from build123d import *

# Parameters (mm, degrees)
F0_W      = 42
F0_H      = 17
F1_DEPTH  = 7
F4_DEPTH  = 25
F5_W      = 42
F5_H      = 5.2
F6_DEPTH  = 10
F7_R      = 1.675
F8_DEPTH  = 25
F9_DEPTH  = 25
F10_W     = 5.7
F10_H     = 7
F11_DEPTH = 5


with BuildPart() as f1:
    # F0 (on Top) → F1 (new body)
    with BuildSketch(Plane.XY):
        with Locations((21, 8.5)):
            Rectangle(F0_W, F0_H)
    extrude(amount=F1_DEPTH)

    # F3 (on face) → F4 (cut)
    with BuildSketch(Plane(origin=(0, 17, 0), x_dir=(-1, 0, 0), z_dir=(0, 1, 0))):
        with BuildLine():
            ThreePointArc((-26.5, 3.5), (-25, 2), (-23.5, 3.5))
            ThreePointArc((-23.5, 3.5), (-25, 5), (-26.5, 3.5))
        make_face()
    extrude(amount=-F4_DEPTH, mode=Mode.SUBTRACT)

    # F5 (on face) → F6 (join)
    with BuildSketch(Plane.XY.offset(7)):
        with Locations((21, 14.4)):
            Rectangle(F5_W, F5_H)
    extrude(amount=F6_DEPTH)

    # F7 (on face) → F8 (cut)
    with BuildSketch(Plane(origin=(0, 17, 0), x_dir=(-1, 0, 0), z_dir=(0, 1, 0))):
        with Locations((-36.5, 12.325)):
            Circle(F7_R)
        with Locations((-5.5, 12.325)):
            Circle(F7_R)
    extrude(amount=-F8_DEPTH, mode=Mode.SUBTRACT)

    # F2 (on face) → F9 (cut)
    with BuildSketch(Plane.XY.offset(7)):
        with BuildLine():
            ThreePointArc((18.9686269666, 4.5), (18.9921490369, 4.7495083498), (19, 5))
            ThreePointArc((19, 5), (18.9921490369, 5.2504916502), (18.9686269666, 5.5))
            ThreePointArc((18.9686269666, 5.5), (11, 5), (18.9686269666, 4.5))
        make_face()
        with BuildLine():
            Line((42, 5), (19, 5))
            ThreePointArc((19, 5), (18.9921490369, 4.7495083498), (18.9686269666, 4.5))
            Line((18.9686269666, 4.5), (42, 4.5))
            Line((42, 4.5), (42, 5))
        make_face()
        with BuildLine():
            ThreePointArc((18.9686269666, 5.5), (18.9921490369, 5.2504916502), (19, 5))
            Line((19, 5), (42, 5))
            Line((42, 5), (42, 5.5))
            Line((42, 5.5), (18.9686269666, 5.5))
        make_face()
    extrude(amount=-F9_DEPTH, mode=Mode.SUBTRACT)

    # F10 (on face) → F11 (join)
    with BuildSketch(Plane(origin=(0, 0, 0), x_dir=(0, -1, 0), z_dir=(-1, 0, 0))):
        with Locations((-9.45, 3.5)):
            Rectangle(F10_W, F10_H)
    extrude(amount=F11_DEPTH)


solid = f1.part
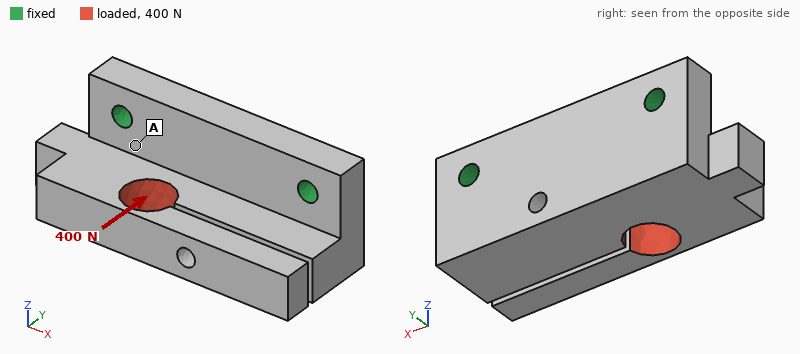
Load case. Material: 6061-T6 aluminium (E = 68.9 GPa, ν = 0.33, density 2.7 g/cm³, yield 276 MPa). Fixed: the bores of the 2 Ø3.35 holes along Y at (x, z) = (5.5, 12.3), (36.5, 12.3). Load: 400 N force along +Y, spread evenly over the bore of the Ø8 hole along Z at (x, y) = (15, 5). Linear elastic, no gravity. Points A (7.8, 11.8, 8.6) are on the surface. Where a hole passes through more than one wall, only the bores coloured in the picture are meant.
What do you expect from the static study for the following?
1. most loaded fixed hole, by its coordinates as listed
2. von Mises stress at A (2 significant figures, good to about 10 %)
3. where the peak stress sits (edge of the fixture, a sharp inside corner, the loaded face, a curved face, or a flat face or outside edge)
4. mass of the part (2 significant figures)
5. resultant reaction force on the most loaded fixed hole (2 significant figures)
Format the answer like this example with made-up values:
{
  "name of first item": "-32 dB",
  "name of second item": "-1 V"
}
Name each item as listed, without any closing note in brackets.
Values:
{
  "most loaded fixed hole, by its coordinates as listed": "(5.5, 12.3)",
  "von Mises stress at A": "23 MPa",
  "where the peak stress sits": "the loaded face",
  "mass of the part": "18 g",
  "resultant reaction force on the most loaded fixed hole": "290 N"
}
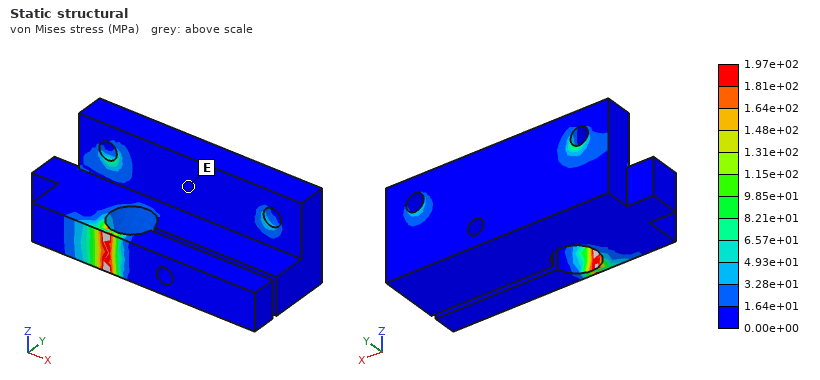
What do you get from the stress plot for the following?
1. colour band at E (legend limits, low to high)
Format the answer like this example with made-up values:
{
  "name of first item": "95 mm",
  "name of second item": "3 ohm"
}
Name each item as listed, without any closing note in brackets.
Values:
{
  "colour band at E": "0.00e+00 to 1.64e+01 MPa"
}
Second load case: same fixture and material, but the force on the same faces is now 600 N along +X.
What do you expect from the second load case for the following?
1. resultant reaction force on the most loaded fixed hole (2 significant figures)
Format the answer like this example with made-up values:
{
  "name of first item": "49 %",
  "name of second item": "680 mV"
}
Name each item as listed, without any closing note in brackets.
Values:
{
  "resultant reaction force on the most loaded fixed hole": "370 N"
}
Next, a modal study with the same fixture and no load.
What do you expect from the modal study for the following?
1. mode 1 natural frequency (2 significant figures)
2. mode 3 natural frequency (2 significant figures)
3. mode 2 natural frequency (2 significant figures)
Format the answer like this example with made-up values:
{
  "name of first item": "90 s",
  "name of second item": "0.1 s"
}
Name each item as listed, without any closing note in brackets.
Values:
{
  "mode 1 natural frequency": "740 Hz",
  "mode 3 natural frequency": "7800 Hz",
  "mode 2 natural frequency": "2600 Hz"
}
